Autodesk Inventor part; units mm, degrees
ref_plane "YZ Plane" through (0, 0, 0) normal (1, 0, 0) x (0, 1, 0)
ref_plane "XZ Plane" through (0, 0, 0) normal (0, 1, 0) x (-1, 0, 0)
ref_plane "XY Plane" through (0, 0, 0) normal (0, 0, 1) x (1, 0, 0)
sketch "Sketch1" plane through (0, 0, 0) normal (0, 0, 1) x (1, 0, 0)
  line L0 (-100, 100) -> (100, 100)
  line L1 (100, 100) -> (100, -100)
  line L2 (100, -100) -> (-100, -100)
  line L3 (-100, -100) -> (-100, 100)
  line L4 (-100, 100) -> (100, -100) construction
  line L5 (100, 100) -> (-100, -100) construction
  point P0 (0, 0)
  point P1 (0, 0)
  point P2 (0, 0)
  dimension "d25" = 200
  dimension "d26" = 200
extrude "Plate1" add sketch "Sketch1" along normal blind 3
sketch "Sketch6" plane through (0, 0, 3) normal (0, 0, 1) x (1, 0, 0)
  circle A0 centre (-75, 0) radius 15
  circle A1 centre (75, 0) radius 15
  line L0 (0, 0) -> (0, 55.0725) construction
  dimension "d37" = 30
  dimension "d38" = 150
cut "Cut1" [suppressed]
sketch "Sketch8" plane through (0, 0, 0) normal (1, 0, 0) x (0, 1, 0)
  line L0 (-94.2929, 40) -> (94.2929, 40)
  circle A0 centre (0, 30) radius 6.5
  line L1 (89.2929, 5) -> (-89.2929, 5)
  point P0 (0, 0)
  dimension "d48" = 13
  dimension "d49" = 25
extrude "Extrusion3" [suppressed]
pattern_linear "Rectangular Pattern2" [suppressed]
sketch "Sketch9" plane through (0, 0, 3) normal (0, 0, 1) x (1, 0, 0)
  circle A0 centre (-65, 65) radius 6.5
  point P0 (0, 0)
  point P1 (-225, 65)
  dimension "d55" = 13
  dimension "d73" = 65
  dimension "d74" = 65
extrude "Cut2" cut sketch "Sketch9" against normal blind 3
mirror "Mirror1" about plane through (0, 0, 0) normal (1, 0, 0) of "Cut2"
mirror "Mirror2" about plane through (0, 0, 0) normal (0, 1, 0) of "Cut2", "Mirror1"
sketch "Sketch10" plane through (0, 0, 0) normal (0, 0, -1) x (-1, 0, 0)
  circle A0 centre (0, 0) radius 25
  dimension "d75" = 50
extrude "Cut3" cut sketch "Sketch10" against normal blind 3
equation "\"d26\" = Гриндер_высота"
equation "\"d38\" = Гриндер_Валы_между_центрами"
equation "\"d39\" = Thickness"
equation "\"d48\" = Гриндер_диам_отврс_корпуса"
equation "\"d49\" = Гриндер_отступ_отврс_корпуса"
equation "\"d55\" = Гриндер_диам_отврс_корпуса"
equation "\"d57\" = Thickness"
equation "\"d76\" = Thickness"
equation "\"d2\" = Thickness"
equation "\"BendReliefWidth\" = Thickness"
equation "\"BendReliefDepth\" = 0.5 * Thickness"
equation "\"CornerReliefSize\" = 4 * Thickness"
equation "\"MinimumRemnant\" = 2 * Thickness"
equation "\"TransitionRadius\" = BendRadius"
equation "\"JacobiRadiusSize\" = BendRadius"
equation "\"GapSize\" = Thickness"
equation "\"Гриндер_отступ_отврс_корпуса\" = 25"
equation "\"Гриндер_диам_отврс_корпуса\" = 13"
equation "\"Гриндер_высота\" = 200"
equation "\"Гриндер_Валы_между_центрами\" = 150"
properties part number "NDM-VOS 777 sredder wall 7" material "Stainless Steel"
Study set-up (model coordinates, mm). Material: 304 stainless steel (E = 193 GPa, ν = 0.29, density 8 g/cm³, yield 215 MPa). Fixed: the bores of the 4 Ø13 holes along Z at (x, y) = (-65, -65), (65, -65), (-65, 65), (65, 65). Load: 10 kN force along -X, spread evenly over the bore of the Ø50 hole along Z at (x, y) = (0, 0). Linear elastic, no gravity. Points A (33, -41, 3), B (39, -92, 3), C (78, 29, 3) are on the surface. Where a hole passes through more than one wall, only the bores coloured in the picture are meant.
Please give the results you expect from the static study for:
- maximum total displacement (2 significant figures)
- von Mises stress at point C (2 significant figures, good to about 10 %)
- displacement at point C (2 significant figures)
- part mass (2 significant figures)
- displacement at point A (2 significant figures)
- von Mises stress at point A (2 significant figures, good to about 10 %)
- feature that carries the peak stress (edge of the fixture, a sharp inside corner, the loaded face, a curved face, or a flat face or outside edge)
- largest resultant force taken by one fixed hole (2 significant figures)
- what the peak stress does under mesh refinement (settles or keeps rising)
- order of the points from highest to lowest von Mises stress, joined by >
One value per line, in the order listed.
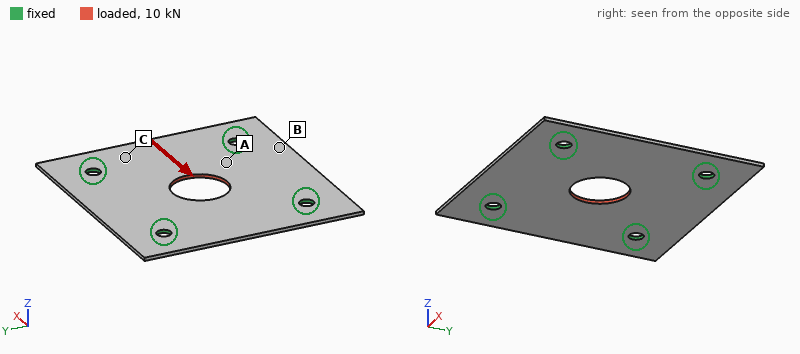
9.6 µm
9.7 MPa
4.9 µm
900 g
4.5 µm
18 MPa
edge of the fixture
2.7 kN
keeps rising
A > C > B
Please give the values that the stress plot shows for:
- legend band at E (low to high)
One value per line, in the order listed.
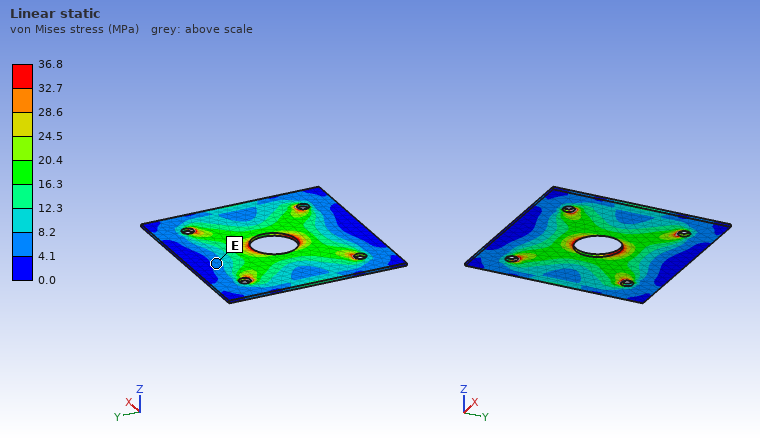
4.1 to 8.2 MPa
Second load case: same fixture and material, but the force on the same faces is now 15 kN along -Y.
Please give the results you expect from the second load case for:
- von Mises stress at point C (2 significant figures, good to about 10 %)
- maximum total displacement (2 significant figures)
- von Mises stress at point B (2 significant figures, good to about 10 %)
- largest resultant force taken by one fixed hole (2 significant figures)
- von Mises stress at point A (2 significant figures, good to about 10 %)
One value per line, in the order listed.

8.2 MPa
14 µm
11 MPa
4.0 kN
27 MPa
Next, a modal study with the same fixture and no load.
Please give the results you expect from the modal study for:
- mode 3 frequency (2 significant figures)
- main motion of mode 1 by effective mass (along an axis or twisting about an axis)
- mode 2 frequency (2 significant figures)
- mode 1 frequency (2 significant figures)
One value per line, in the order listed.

960 Hz
along Z
930 Hz
750 Hz
